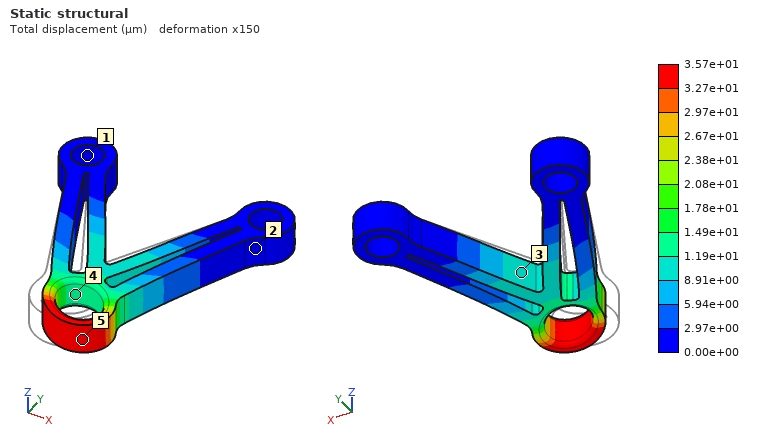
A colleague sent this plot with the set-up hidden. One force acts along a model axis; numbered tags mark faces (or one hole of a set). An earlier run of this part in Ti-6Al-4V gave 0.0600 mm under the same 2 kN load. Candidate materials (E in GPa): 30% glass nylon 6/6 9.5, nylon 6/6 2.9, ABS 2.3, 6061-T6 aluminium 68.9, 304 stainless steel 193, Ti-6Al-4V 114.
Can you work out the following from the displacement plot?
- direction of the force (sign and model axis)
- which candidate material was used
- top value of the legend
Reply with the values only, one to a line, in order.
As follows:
+X
304 stainless steel
3.57e+01 µm
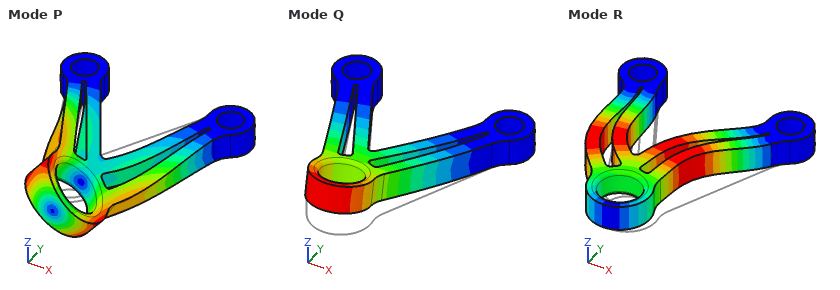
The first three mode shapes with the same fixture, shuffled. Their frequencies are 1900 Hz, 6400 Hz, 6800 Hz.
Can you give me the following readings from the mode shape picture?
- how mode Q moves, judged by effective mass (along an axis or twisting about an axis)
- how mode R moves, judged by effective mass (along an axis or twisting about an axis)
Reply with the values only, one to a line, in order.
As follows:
along Z
along X
